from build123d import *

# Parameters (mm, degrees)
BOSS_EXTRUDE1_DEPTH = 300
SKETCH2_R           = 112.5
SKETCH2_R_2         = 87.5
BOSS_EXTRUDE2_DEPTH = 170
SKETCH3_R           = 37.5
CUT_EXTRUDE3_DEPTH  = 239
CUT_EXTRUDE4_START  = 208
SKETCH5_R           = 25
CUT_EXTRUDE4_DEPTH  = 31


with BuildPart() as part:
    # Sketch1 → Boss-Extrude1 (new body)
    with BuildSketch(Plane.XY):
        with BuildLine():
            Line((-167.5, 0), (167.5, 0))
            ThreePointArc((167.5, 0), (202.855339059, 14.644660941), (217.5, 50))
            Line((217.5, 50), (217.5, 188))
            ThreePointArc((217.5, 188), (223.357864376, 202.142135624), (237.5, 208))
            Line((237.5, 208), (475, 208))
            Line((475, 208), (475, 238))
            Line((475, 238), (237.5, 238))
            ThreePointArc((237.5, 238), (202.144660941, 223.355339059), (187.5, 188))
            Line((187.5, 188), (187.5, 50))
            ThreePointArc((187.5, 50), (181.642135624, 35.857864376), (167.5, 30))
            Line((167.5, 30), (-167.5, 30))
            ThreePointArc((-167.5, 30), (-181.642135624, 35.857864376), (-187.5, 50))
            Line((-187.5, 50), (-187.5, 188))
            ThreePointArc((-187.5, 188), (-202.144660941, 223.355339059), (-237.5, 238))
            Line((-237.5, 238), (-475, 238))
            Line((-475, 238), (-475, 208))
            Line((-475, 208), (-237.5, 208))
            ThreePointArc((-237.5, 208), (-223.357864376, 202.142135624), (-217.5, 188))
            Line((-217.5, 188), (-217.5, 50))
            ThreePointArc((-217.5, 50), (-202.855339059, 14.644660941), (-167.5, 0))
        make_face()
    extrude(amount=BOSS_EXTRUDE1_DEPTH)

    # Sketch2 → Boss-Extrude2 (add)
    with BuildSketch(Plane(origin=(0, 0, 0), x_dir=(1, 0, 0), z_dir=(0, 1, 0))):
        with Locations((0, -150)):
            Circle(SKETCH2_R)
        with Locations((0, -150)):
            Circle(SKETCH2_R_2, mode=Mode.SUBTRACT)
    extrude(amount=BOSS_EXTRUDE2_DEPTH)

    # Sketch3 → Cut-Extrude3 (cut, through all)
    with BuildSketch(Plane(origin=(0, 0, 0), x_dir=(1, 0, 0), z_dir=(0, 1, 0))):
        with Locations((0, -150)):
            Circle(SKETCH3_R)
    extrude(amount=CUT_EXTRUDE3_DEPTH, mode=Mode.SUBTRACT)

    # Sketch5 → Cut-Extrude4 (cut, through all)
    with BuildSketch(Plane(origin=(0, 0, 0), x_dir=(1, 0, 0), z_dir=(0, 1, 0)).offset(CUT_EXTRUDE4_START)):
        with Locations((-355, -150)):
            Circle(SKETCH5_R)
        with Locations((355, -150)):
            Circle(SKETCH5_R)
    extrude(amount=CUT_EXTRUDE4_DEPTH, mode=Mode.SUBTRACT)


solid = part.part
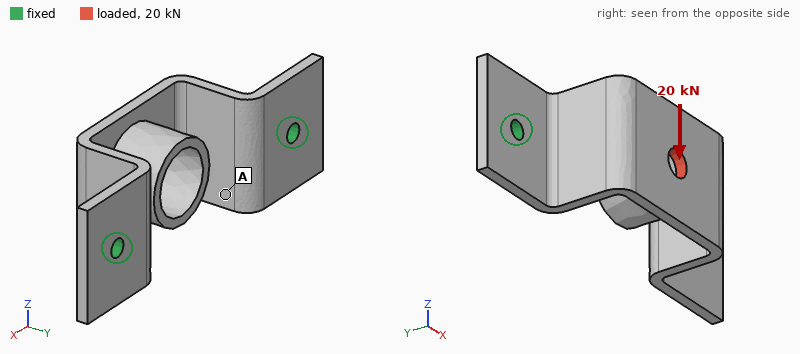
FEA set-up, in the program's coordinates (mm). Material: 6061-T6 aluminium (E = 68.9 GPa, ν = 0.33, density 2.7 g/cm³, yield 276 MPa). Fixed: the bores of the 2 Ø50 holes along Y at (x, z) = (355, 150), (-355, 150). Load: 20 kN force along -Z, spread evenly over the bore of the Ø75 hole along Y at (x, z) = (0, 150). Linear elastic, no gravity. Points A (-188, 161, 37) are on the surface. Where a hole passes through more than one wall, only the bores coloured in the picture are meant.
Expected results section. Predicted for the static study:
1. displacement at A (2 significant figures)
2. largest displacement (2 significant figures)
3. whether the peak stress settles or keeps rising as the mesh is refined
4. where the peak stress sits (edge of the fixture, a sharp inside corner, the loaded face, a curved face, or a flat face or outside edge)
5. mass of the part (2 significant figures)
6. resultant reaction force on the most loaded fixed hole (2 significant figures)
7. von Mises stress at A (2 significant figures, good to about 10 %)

0.46 mm
0.96 mm
keeps rising
edge of the fixture
37 kg
10 kN
10 MPa
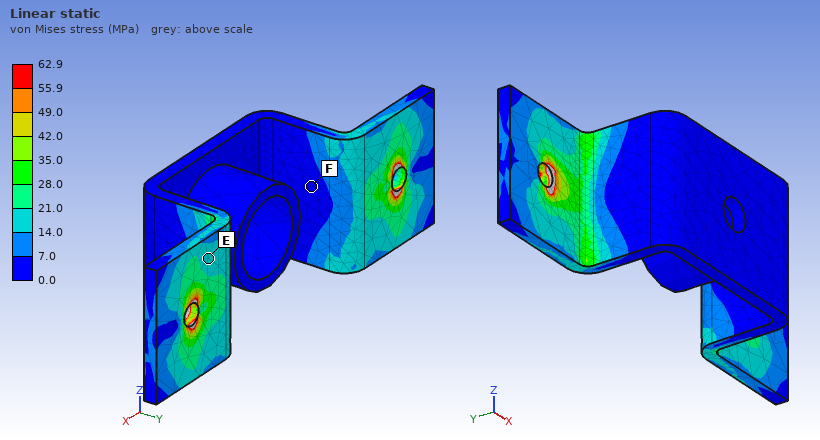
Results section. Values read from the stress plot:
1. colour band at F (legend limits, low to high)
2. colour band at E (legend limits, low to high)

0.0 to 7.0 MPa
14.0 to 21.0 MPa
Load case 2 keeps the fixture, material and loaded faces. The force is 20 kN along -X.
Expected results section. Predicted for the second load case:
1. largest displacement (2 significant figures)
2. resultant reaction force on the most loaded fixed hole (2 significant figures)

0.50 mm
12 kN
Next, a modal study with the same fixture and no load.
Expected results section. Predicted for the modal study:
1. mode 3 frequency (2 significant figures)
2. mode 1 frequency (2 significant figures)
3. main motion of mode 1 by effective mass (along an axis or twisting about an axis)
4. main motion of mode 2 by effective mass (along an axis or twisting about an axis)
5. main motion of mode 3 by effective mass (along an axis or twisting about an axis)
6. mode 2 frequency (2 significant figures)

400 Hz
190 Hz
along Z
along X
along Y
240 Hz
